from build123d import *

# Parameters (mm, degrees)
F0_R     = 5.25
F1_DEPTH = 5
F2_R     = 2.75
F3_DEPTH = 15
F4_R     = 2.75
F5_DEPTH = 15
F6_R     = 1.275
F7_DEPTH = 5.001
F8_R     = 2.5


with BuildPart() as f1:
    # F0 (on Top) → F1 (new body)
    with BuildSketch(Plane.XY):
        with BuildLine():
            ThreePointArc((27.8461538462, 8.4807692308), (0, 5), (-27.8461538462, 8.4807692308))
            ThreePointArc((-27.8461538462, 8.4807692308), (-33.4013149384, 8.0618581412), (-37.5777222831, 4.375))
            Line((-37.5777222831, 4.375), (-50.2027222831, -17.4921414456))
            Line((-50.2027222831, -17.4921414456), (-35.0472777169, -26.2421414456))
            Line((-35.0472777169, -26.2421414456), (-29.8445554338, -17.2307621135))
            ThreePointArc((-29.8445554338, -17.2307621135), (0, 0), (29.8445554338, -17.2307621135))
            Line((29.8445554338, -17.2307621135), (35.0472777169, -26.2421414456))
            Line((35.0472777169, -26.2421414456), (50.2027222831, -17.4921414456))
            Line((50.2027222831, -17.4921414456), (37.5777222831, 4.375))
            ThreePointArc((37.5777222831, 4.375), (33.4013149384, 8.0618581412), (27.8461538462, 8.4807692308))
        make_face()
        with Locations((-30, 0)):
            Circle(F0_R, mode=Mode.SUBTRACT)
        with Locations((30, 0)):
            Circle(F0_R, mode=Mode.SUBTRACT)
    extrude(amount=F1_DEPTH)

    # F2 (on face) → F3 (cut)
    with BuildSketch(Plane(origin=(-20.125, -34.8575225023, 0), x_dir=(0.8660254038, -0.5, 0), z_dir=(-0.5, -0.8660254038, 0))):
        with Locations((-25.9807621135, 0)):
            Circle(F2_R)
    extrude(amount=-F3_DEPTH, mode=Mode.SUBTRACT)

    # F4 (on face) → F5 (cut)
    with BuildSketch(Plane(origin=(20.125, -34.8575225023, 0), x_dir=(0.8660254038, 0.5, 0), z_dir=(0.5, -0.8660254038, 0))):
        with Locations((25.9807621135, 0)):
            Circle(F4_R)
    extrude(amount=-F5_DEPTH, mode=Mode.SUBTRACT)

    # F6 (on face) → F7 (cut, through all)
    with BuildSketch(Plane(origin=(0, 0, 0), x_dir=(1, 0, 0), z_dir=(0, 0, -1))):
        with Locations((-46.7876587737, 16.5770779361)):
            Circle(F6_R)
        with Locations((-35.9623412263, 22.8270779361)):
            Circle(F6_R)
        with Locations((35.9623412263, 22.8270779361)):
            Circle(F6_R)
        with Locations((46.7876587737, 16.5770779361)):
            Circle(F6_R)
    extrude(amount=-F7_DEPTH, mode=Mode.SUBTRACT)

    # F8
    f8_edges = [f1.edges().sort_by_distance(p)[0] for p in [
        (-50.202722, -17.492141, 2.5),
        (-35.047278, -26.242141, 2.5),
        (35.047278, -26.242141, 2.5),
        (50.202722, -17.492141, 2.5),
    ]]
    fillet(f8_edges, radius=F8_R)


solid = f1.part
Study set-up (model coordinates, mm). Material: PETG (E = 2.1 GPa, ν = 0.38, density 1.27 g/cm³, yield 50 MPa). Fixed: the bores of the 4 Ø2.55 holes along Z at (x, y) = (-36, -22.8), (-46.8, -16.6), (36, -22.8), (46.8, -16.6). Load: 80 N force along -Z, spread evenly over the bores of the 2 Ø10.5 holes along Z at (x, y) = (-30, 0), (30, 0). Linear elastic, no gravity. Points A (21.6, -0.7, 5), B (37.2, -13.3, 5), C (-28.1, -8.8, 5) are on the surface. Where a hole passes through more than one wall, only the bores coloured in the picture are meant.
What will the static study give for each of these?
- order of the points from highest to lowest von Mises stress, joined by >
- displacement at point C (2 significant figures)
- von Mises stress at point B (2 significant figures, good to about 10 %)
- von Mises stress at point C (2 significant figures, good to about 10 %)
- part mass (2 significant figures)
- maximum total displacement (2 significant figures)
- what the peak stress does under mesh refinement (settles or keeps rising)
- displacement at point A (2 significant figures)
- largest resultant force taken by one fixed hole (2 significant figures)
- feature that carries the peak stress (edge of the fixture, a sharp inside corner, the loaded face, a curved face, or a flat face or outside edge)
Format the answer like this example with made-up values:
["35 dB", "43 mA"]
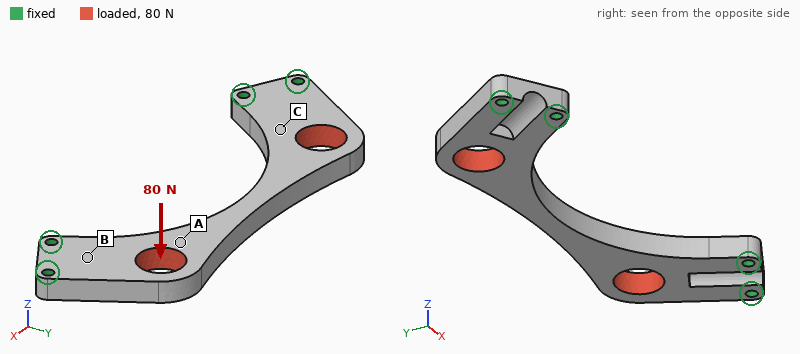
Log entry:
["B > C > A", "0.27 mm", "7.5 MPa", "4.3 MPa", "7.9 g", "0.84 mm", "keeps rising", "0.56 mm", "26 N", "edge of the fixture"]
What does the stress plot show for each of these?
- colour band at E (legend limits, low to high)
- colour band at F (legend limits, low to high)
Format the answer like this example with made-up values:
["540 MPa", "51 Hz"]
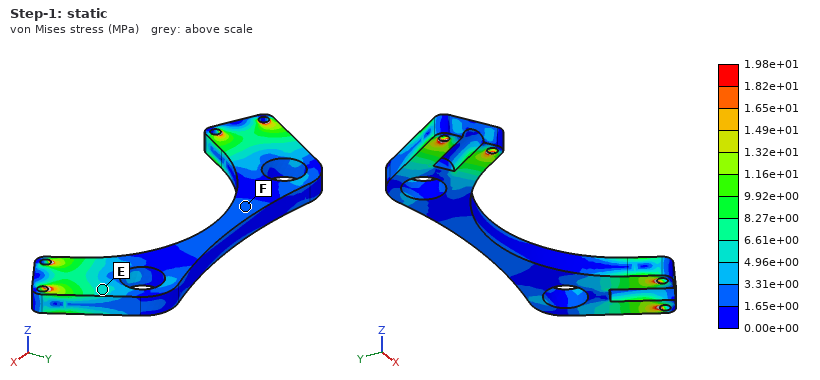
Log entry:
["4.96e+00 to 6.61e+00 MPa", "1.65e+00 to 3.31e+00 MPa"]
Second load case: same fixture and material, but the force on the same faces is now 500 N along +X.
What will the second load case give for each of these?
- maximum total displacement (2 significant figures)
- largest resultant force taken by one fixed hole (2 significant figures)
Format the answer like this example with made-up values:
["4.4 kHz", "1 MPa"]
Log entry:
["0.27 mm", "320 N"]
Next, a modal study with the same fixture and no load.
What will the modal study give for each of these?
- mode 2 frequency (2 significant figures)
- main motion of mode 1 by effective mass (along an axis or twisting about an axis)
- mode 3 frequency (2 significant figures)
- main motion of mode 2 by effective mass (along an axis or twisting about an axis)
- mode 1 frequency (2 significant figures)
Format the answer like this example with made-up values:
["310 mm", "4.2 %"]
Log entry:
["1400 Hz", "along Z", "2200 Hz", "twisting about Y", "690 Hz"]
